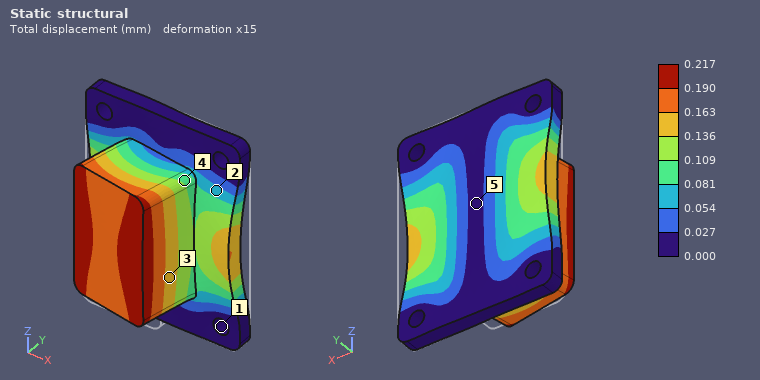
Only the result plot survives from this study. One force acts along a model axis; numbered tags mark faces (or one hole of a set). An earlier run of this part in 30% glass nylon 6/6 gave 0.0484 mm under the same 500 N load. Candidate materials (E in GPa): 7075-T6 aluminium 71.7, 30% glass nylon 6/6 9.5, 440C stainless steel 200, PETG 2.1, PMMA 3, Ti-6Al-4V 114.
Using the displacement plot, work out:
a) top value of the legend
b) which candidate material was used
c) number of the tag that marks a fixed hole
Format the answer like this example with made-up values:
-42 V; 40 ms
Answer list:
0.217 mm; PETG; 1
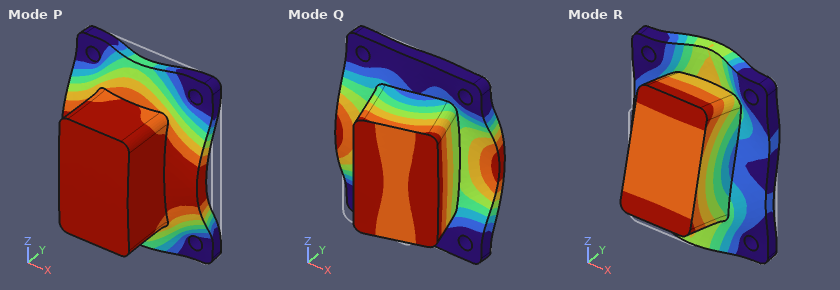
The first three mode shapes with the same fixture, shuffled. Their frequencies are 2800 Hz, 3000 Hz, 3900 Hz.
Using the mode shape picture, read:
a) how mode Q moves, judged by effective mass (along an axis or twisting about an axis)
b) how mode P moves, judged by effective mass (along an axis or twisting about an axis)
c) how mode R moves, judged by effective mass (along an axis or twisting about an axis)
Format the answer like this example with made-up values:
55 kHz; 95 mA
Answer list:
along X; along Y; along Z
